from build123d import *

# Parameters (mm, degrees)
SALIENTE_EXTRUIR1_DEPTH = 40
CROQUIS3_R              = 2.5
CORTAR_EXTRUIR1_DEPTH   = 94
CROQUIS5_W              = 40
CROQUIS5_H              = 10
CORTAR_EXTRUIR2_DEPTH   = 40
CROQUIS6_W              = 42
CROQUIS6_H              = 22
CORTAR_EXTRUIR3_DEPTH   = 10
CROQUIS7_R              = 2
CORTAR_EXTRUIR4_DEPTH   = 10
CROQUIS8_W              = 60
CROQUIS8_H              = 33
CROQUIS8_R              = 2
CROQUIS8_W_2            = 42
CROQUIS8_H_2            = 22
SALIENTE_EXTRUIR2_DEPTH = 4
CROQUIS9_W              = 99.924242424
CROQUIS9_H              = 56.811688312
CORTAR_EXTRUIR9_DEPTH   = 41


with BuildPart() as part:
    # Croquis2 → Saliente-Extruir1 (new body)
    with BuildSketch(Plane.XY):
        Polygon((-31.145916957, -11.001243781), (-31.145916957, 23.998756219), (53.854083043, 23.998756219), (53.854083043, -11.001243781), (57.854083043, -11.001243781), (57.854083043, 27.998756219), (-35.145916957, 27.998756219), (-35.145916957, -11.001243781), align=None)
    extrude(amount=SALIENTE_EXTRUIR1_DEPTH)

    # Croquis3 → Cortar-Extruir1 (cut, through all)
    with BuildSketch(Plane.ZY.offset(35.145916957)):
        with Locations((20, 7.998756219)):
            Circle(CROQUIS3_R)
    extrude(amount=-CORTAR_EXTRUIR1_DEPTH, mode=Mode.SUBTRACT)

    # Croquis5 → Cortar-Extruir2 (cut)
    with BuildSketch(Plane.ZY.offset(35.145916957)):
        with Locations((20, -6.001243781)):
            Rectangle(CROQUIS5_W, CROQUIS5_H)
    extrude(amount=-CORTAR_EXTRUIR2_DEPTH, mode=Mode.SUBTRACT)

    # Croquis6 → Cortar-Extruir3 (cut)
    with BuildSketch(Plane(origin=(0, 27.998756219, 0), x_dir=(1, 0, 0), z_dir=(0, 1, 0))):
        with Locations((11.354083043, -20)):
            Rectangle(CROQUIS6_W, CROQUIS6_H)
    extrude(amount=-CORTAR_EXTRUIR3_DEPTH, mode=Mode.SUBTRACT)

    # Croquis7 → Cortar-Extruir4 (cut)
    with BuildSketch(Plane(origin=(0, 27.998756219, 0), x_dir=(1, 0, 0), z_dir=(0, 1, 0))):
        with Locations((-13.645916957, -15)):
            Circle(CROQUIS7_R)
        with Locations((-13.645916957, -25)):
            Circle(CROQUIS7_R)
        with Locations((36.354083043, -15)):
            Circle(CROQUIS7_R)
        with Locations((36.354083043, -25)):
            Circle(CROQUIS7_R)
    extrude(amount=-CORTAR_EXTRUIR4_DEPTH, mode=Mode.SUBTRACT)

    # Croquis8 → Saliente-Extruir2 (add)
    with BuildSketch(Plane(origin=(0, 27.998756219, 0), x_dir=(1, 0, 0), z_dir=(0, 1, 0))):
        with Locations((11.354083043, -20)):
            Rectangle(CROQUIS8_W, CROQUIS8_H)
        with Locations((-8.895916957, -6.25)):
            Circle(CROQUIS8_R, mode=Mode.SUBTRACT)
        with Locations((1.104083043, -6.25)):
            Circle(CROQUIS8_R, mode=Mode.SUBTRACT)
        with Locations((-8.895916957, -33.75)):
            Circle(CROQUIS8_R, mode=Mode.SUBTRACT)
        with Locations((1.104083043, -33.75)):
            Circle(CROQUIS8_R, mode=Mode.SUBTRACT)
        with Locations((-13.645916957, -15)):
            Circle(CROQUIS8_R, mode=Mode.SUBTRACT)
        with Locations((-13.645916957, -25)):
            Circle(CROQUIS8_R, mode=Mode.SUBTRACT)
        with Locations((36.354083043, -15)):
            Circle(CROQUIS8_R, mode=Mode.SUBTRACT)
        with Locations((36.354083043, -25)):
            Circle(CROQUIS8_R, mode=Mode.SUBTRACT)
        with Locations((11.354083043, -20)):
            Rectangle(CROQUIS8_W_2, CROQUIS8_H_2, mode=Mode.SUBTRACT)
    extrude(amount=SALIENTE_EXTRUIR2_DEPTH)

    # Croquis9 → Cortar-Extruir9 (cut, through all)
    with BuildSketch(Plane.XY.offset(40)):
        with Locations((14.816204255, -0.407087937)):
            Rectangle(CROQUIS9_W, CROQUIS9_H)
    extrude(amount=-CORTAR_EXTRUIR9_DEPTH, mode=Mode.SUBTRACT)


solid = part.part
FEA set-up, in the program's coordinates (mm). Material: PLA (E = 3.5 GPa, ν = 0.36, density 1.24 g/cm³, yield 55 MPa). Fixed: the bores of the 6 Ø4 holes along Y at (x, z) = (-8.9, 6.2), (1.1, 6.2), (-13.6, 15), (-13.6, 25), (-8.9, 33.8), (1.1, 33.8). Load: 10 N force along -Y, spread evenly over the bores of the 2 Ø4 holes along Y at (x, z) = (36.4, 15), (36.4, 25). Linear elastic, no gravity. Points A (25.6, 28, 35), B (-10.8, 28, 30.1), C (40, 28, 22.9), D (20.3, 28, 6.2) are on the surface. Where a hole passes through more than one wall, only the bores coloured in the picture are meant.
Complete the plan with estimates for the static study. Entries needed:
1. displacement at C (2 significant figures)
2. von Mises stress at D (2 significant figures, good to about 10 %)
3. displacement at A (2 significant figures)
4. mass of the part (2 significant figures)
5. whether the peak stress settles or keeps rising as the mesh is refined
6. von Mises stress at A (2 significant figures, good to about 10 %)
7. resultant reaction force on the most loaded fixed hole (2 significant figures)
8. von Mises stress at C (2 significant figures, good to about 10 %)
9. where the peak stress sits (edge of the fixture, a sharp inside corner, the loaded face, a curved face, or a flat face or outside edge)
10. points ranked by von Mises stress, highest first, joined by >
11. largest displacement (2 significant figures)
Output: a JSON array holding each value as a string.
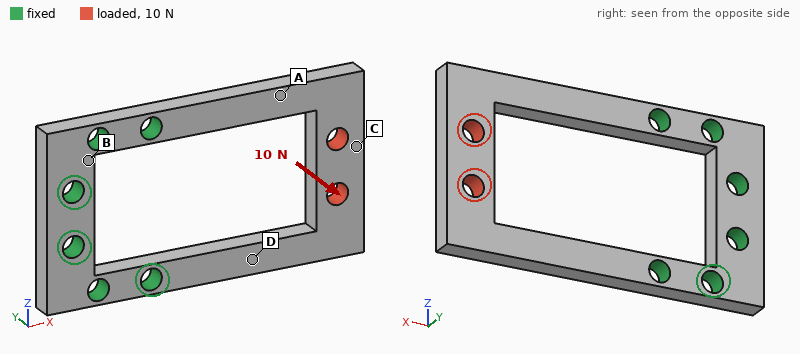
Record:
["0.75 mm", "5.5 MPa", "0.34 mm", "4.7 g", "keeps rising", "3.7 MPa", "5.1 N", "2.2 MPa", "edge of the fixture", "D > A > C > B", "0.79 mm"]
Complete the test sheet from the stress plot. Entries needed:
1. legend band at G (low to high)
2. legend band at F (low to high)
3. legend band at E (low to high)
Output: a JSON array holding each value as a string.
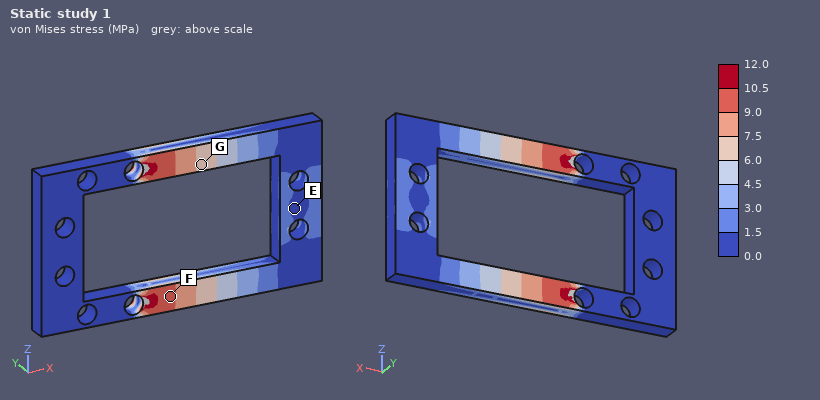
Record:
["6.0 to 7.5 MPa", "9.0 to 10.5 MPa", "0.0 to 1.5 MPa"]
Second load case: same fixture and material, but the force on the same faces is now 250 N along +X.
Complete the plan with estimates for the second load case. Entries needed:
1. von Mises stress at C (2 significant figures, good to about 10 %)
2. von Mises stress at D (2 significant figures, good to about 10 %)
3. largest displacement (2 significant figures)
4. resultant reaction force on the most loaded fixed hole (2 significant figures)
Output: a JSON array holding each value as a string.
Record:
["12 MPa", "5.9 MPa", "0.17 mm", "130 N"]
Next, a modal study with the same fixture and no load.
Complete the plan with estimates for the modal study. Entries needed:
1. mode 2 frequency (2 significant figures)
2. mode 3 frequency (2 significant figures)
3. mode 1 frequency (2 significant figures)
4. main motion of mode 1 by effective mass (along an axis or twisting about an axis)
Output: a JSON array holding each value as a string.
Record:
["1200 Hz", "1200 Hz", "490 Hz", "along Y"]
